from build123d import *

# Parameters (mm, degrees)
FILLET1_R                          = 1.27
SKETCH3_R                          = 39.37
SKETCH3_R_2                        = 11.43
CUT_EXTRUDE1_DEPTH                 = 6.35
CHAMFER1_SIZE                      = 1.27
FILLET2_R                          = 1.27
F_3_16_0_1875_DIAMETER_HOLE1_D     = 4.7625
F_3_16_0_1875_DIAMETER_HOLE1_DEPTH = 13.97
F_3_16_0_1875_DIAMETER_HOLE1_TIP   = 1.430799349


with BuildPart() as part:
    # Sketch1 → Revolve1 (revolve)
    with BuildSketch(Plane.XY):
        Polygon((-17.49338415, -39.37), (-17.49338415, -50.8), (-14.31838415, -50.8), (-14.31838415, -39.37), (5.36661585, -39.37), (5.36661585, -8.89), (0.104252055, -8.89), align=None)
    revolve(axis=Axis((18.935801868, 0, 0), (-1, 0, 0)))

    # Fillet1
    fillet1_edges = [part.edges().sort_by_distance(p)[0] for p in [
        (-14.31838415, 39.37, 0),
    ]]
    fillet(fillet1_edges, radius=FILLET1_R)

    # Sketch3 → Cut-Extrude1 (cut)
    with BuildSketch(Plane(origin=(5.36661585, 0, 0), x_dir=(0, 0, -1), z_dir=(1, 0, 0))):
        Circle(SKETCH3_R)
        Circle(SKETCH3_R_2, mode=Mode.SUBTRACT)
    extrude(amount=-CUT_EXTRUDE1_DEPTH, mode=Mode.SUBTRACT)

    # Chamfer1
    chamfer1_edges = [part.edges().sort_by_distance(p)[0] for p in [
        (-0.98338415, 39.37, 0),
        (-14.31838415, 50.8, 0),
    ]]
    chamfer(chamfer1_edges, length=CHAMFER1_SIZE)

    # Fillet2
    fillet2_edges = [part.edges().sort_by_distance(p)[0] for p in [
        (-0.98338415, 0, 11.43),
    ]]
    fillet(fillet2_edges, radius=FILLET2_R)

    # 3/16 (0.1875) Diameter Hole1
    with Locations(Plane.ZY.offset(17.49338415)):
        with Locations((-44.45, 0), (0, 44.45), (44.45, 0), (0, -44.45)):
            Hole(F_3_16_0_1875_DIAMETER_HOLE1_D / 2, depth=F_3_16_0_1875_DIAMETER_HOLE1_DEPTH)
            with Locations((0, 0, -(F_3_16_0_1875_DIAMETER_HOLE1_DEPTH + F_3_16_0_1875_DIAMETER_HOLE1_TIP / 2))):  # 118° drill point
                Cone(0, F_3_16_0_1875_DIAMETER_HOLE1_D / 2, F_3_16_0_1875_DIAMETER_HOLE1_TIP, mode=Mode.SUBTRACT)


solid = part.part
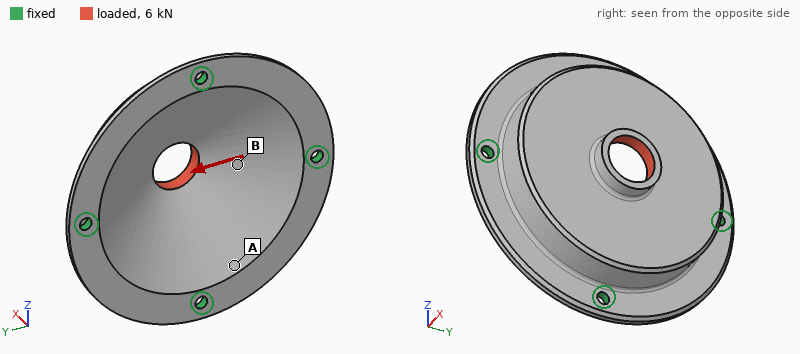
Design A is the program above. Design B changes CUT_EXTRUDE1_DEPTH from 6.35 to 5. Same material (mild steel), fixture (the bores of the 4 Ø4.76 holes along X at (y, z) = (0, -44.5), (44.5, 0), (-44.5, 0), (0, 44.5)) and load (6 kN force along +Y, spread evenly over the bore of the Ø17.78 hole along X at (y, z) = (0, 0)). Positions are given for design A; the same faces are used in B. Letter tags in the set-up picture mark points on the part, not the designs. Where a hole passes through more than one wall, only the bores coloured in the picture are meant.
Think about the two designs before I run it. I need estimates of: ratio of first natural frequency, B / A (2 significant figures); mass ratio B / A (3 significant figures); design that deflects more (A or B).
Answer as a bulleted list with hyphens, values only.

- 0.97
- 1.11
- A
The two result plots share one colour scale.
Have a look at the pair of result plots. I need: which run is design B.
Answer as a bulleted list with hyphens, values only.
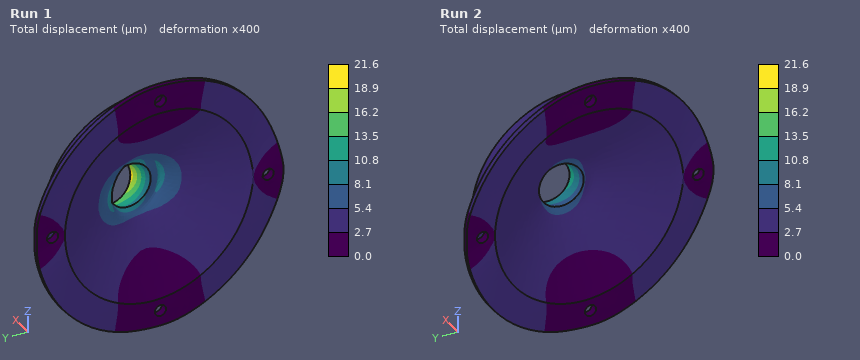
- Run 2
